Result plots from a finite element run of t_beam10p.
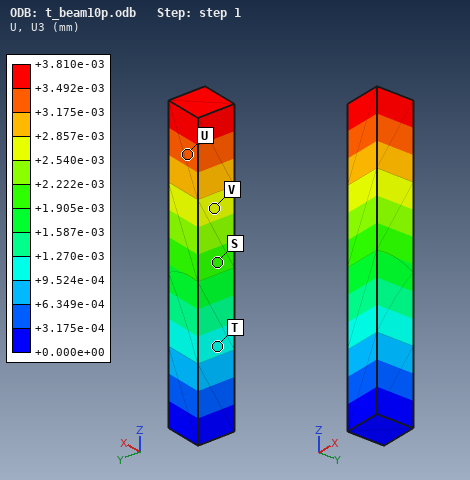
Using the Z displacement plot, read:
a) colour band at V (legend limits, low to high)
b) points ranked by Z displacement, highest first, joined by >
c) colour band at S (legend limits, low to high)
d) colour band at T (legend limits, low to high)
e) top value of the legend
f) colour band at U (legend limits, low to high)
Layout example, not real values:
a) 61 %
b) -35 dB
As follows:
a) +2.540e-03 to +2.857e-03 mm
b) U > V > S > T
c) +1.905e-03 to +2.222e-03 mm
d) +9.524e-04 to +1.270e-03 mm
e) +3.810e-03 mm
f) +3.175e-03 to +3.492e-03 mm
